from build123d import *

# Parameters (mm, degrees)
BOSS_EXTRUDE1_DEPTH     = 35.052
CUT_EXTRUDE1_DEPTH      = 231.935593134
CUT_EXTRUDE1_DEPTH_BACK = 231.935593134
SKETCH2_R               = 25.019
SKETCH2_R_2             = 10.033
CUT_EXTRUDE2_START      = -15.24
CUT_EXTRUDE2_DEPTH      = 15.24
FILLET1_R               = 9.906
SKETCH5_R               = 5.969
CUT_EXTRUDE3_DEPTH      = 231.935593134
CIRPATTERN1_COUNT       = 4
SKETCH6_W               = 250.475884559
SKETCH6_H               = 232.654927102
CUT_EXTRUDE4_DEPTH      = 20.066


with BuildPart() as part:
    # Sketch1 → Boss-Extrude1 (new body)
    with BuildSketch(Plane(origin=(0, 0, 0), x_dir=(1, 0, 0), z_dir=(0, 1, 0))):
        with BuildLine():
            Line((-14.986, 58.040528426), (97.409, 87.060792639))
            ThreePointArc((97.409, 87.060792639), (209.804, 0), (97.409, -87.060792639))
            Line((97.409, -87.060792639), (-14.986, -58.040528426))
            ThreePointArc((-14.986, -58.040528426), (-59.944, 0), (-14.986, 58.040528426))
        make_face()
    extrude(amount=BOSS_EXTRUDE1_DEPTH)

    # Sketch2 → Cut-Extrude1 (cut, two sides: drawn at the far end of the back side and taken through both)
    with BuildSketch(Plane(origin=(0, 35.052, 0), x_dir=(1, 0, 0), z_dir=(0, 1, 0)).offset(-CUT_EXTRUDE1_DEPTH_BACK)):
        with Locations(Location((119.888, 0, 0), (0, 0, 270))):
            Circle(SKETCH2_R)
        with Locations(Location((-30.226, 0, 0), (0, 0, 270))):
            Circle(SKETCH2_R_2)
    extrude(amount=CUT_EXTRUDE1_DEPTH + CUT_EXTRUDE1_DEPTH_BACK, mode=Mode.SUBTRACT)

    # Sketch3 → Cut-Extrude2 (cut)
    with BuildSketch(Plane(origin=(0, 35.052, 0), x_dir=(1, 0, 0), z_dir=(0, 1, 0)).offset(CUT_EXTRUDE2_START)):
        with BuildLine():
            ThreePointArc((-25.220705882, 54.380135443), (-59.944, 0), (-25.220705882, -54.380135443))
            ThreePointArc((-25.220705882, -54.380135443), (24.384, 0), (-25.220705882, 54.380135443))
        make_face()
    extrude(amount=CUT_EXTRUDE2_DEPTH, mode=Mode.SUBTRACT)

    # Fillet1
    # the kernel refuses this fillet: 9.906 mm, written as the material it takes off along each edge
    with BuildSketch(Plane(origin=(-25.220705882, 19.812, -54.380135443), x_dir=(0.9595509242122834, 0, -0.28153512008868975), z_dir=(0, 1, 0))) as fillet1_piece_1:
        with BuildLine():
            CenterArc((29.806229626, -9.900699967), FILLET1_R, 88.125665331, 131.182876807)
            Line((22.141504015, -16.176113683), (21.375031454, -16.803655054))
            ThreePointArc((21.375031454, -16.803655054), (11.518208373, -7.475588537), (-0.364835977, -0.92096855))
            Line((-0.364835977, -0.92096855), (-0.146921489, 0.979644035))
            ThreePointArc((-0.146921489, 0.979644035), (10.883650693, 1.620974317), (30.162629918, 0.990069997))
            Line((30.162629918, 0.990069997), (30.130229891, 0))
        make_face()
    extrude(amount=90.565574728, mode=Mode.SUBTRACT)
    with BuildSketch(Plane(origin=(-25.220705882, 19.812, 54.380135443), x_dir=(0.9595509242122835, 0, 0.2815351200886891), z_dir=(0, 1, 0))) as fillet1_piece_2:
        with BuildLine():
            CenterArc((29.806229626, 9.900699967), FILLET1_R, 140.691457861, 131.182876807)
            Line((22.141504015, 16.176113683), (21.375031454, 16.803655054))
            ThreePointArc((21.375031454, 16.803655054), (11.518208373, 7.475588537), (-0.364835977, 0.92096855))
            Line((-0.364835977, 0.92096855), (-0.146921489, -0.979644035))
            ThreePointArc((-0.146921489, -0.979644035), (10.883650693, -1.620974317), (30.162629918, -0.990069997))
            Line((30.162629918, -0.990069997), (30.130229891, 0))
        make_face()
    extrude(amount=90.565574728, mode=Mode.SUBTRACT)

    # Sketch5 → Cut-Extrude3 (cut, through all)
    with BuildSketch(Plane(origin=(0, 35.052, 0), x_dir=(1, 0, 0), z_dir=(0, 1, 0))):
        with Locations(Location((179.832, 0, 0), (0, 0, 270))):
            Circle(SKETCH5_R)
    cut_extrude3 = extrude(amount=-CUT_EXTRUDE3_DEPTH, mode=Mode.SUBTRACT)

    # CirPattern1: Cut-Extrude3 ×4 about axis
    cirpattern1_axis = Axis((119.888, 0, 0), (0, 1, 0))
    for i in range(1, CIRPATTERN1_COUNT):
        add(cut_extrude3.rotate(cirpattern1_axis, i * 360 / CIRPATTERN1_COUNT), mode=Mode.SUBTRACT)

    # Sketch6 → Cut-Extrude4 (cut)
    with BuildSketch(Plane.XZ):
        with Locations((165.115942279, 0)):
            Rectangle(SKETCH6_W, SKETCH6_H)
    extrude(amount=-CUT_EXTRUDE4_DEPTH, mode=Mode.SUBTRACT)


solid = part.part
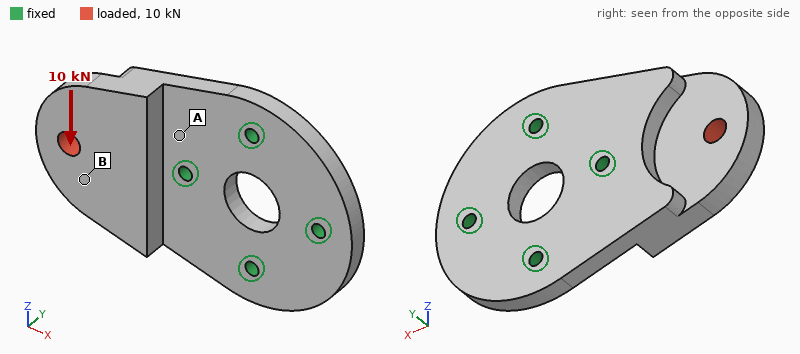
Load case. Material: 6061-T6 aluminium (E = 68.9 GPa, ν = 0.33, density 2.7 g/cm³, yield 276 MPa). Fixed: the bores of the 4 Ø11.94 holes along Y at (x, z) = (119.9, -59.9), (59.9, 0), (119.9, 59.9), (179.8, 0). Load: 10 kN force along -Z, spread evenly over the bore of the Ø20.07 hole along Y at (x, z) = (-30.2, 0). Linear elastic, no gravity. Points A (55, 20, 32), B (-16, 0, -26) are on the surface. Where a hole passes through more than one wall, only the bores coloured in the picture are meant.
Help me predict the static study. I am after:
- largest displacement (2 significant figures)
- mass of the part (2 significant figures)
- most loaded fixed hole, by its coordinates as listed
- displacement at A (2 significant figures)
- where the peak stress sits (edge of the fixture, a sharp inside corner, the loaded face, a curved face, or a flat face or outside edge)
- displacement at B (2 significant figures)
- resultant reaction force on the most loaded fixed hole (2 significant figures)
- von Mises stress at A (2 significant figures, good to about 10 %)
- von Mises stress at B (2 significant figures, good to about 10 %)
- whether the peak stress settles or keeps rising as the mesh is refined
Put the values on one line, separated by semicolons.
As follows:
70 µm; 1.7 kg; (59.9, 0); 19 µm; edge of the fixture; 53 µm; 10 kN; 14 MPa; 5.2 MPa; keeps rising
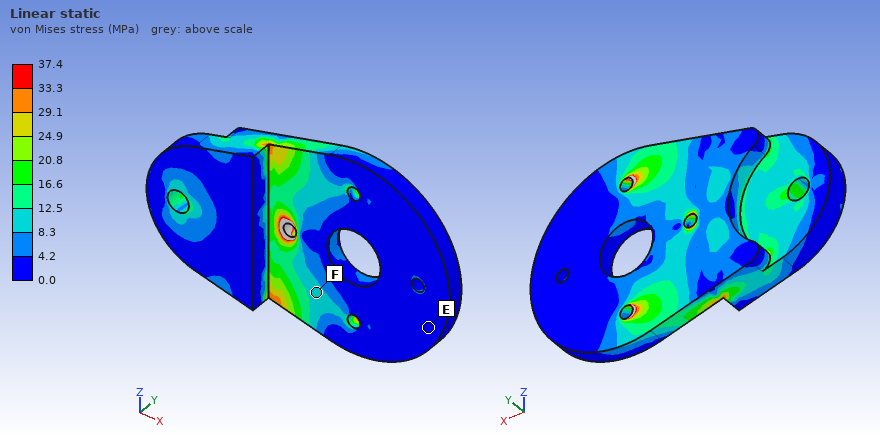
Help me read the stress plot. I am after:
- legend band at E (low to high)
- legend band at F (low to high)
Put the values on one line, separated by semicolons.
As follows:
0.0 to 4.2 MPa; 8.3 to 12.5 MPa
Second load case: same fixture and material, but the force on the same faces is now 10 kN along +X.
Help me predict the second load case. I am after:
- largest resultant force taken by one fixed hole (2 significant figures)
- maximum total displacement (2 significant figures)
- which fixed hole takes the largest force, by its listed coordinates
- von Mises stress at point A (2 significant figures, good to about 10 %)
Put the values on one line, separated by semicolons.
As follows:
5.4 kN; 0.23 mm; (59.9, 0); 25 MPa
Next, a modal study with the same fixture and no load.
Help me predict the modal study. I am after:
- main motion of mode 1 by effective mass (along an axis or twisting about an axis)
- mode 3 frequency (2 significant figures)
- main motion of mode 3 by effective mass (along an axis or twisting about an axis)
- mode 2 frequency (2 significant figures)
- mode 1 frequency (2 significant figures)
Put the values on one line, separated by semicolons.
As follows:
along Y; 3400 Hz; along Z; 1700 Hz; 920 Hz
